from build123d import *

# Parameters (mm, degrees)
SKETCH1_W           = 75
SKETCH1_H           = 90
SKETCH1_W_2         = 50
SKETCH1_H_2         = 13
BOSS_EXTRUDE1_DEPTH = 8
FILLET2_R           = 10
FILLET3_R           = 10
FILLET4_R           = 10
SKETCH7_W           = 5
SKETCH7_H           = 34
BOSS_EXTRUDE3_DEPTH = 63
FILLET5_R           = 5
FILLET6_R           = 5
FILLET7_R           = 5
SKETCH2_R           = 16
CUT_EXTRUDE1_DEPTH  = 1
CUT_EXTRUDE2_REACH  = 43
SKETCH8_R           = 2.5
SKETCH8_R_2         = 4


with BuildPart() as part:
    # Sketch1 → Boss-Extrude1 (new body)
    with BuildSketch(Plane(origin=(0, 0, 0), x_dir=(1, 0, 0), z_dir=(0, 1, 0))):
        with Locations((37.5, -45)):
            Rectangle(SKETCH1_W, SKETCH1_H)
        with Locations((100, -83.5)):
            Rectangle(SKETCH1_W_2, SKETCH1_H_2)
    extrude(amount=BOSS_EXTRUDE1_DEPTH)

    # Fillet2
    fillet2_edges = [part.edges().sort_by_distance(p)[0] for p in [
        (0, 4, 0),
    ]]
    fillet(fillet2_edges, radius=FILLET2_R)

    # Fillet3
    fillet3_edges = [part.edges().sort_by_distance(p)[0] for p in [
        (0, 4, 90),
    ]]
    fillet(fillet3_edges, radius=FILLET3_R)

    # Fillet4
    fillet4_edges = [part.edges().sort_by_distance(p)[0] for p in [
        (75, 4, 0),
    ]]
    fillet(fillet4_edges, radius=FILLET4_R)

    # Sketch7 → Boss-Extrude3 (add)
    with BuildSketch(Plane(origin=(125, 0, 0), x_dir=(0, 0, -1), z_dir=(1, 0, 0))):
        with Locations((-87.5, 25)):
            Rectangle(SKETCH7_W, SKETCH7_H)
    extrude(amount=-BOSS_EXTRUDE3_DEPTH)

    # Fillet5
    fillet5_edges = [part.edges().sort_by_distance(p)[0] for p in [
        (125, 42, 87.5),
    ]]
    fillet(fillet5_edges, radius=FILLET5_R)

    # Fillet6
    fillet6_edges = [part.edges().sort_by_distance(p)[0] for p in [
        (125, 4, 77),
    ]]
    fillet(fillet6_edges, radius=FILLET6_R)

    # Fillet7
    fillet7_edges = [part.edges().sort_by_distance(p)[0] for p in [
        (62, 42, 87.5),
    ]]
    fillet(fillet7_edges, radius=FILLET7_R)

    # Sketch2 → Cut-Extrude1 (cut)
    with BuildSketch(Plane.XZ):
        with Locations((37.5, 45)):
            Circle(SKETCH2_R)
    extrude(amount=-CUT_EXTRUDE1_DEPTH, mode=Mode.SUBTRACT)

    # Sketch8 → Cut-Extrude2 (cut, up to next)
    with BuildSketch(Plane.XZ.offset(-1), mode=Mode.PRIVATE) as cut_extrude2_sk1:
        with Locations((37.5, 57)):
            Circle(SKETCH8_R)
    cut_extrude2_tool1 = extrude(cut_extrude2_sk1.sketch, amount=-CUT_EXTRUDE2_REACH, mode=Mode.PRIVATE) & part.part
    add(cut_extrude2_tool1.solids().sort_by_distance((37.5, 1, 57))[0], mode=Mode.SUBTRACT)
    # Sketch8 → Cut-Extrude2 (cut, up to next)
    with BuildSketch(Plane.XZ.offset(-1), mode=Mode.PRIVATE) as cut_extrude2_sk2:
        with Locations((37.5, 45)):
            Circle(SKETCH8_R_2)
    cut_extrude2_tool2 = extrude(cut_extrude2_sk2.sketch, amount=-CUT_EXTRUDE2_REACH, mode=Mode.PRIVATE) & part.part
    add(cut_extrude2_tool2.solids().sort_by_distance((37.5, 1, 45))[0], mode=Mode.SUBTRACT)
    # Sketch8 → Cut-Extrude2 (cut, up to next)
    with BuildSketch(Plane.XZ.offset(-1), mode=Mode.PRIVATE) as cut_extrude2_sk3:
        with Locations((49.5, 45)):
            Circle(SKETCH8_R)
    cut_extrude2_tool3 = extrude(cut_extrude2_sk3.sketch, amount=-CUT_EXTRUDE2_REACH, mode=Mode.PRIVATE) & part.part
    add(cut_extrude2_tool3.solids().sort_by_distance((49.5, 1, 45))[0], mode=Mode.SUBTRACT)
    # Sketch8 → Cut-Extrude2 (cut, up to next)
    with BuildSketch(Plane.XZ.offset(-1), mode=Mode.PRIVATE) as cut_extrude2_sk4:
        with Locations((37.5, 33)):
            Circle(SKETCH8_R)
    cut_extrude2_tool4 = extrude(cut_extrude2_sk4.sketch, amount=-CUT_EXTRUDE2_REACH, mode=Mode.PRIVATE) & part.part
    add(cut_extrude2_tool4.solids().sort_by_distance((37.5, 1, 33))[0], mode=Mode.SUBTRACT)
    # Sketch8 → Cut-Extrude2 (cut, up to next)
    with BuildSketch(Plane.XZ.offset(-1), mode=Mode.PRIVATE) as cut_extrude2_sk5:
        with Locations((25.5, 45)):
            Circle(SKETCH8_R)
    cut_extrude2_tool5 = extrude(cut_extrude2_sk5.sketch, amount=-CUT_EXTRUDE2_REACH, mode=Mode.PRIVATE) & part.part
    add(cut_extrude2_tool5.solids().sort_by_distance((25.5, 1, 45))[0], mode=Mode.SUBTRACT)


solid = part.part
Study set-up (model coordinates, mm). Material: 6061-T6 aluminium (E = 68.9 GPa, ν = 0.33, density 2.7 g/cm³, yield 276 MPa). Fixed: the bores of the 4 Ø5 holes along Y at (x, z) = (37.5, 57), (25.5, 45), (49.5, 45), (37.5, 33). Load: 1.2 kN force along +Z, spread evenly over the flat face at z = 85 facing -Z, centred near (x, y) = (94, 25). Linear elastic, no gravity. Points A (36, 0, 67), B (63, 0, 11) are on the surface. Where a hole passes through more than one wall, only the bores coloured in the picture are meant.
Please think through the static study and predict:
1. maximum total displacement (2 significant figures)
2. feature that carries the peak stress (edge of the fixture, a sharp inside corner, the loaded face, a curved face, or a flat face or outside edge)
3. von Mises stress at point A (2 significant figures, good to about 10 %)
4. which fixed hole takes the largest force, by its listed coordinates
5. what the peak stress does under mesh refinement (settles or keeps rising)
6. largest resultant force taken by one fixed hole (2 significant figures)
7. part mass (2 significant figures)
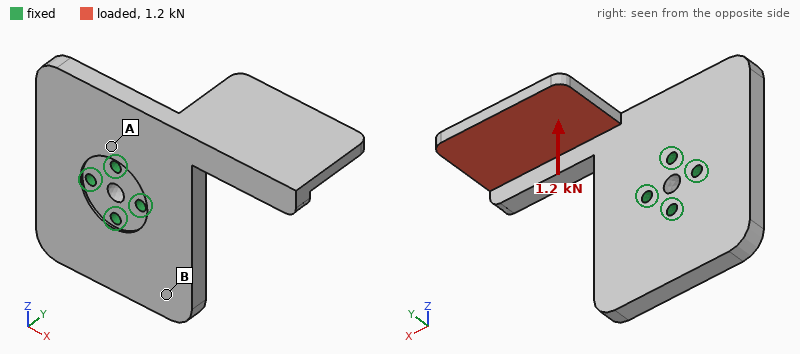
1.0 mm
a sharp inside corner
39 MPa
(49.5, 45)
keeps rising
2.0 kN
180 g
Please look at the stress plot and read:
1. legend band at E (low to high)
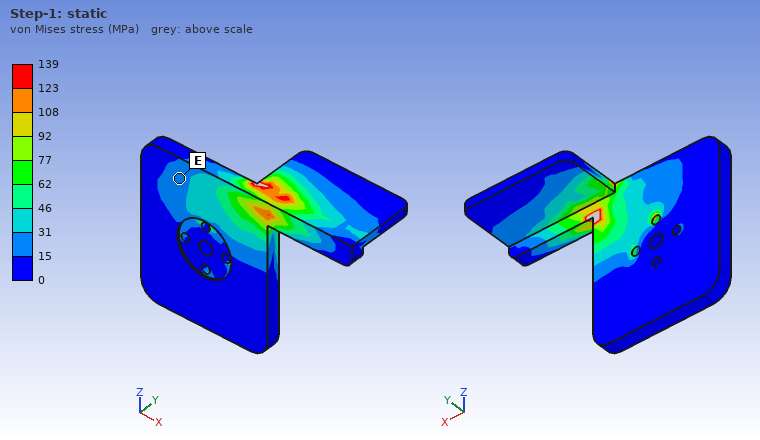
15 to 31 MPa
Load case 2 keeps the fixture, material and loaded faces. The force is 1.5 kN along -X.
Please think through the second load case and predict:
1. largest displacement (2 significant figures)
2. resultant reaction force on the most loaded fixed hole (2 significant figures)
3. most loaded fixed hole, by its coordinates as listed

0.90 mm
1.9 kN
(37.5, 57)
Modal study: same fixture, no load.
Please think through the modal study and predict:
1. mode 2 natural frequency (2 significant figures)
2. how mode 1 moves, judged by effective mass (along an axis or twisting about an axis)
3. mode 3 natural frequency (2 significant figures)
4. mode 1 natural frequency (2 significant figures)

1500 Hz
along Y
2600 Hz
790 Hz
